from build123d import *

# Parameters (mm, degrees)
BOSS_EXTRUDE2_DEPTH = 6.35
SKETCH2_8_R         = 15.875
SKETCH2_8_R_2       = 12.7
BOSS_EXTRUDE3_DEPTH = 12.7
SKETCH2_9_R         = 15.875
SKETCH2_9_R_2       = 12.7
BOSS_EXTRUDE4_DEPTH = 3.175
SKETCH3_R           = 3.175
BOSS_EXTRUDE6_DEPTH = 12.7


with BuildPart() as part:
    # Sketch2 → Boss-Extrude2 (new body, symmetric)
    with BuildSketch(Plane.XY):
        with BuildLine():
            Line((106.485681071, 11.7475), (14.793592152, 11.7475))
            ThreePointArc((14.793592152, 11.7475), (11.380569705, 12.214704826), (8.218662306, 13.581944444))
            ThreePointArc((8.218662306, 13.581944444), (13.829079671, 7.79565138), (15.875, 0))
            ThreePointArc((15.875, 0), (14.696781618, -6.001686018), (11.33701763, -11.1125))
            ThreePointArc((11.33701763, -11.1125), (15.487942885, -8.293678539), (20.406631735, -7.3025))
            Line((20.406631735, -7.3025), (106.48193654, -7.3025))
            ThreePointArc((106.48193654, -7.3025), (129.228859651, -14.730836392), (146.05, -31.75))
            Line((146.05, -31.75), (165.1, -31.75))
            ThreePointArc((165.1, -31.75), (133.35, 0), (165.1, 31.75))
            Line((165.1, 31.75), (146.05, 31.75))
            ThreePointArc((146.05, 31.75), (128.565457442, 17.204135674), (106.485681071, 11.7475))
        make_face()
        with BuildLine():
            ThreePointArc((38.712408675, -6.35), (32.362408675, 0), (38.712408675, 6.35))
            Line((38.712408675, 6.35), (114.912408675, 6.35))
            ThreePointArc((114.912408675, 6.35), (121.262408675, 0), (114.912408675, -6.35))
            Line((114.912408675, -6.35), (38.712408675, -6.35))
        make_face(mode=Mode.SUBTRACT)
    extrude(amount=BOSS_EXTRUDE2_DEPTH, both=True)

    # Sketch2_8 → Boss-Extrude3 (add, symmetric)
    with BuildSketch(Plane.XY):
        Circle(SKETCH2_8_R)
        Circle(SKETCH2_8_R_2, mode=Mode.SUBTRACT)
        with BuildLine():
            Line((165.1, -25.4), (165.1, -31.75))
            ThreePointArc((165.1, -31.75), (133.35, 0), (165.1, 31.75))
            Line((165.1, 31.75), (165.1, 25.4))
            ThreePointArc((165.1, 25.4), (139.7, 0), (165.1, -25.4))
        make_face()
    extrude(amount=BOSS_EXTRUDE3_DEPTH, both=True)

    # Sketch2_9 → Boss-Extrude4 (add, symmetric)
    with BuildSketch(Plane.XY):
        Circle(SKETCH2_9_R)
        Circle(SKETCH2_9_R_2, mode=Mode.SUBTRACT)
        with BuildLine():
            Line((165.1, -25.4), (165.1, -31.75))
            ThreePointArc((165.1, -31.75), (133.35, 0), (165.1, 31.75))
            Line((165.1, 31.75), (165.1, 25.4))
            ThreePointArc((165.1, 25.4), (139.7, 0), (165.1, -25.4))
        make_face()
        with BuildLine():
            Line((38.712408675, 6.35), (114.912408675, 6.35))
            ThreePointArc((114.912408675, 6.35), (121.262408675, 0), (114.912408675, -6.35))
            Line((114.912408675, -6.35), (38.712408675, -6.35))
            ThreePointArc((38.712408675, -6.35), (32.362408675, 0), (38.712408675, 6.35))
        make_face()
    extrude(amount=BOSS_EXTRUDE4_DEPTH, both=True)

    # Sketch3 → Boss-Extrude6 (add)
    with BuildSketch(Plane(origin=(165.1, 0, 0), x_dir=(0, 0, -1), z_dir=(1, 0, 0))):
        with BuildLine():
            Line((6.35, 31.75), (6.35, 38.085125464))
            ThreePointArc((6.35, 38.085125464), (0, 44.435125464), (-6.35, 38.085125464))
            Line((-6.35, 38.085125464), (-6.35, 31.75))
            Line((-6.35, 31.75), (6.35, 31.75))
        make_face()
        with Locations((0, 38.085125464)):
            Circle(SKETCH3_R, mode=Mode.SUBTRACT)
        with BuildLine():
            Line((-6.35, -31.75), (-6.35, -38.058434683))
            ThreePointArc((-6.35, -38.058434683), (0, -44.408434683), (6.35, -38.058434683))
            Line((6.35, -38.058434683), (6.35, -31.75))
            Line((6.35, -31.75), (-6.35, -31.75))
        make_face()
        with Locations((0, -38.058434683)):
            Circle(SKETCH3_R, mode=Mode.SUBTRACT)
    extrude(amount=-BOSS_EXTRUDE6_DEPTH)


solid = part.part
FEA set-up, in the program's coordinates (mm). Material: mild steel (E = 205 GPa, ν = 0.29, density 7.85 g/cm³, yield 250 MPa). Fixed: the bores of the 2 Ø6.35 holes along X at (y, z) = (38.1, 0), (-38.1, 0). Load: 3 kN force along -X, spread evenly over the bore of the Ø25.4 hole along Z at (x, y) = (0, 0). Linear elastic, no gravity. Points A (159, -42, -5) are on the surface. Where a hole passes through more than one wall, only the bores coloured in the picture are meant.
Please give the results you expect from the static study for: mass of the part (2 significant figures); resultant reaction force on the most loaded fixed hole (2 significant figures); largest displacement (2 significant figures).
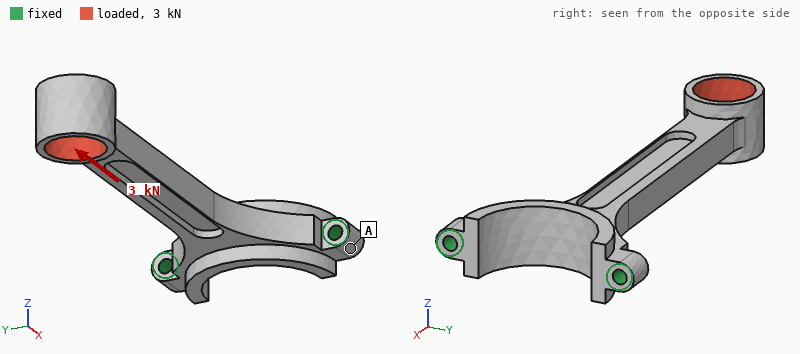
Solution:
410 g
1.9 kN
91 µm
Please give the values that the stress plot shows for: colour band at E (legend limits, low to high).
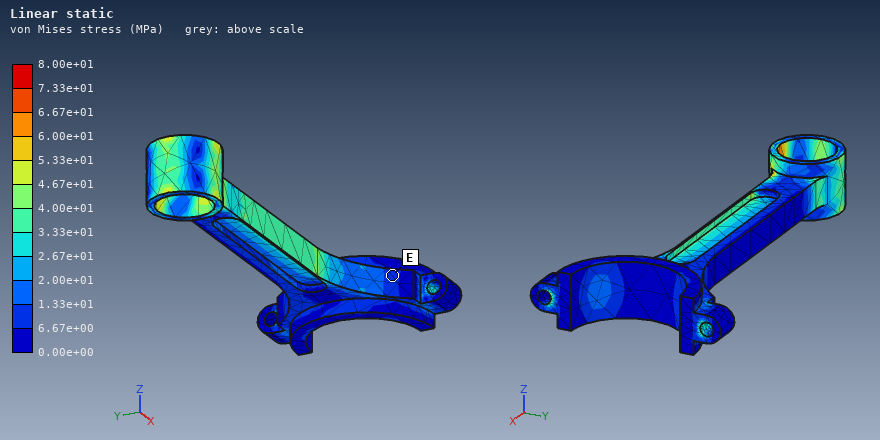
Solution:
6.67e+00 to 1.33e+01 MPa
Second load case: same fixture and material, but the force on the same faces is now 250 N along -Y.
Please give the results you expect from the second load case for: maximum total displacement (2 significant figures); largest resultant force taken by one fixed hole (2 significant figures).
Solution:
0.18 mm
750 N
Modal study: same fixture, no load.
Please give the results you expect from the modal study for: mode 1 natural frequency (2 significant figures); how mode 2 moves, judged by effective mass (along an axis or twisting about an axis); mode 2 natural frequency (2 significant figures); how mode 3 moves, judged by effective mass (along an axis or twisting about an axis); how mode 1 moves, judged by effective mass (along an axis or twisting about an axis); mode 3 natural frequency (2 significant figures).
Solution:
310 Hz
along Y
680 Hz
along Z
along Z
1800 Hz
